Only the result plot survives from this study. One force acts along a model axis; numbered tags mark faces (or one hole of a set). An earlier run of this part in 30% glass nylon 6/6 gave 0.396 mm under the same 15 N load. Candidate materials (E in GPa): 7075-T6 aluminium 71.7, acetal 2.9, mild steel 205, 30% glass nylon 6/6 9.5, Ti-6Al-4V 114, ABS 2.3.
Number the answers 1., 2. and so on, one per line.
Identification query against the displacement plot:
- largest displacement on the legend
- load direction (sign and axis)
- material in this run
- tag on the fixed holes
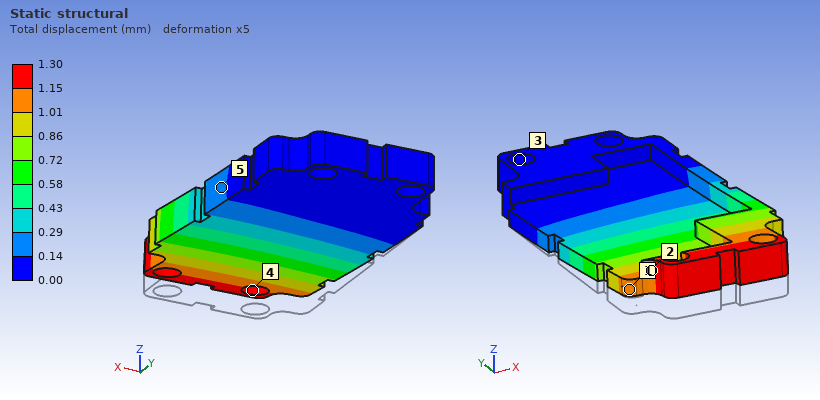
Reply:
1. 1.30 mm
2. +Z
3. acetal
4. 3
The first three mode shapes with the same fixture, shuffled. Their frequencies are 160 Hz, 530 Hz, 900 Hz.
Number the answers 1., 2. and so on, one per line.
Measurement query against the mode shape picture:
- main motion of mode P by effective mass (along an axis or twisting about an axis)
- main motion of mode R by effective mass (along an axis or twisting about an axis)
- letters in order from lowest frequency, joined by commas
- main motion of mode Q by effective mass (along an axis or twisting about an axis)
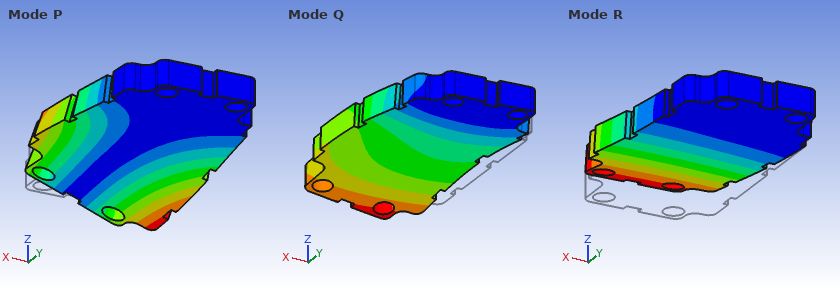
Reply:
1. twisting about Y
2. along Z
3. R, P, Q
4. along X
